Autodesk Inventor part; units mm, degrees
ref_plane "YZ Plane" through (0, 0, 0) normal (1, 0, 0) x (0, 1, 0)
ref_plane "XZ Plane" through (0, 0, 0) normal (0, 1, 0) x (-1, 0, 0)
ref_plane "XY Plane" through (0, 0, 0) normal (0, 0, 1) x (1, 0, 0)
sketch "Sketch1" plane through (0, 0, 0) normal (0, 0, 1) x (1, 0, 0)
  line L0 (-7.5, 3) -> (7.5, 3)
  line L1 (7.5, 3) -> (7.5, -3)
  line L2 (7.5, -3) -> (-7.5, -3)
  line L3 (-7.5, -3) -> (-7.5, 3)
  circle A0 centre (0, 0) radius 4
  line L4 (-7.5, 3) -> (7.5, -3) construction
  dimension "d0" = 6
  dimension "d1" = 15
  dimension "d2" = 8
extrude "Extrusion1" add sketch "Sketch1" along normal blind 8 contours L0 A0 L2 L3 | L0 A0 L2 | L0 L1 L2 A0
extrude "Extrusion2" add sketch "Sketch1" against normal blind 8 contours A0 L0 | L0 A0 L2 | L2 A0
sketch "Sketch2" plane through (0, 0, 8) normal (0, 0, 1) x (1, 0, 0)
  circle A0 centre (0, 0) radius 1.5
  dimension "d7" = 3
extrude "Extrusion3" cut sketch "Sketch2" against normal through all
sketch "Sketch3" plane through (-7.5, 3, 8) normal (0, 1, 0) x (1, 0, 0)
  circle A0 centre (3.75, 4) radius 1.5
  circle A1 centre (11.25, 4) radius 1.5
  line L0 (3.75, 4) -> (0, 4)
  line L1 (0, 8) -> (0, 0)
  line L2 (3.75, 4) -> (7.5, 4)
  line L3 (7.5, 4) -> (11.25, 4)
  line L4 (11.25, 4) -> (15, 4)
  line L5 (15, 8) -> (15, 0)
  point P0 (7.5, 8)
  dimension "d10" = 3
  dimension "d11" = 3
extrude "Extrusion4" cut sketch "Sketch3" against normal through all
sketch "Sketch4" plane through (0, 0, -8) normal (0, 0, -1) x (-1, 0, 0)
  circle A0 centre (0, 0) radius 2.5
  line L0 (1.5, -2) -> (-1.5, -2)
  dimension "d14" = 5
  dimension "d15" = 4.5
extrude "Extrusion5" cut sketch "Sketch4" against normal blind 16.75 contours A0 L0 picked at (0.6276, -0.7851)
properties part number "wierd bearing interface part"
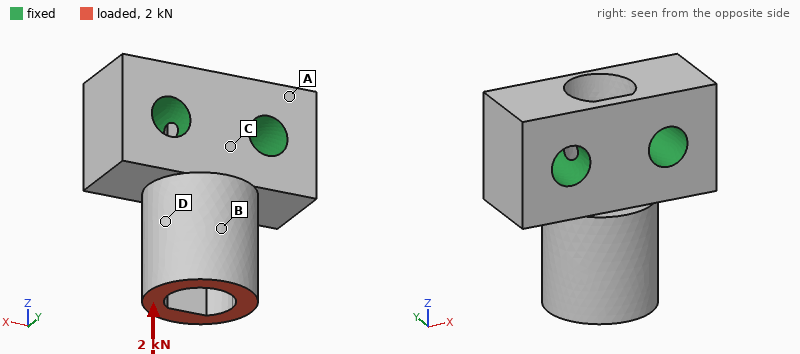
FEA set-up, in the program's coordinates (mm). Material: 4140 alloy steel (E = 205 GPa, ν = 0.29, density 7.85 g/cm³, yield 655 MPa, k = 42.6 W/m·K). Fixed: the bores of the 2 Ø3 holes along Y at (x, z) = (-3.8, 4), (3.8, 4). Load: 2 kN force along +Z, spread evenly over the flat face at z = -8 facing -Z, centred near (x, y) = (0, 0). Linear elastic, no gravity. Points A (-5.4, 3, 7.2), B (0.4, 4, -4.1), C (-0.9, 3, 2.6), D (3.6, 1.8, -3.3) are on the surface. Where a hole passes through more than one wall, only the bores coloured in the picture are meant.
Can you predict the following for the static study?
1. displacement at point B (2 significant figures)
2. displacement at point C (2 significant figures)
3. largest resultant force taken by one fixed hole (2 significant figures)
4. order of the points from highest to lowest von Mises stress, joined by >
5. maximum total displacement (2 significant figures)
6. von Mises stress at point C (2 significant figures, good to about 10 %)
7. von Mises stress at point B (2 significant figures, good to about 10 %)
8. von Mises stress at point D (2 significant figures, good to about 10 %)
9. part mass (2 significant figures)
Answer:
2.5 µm
0.65 µm
1.0 kN
D > B > C > A
3.6 µm
44 MPa
56 MPa
69 MPa
5.8 g
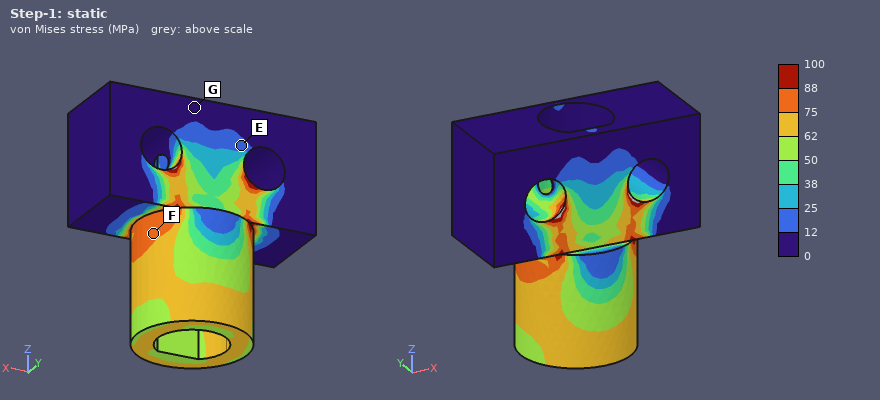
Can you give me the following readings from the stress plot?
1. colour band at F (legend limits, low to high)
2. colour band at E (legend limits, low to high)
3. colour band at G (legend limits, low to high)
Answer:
75 to 88 MPa
12 to 25 MPa
0 to 12 MPa
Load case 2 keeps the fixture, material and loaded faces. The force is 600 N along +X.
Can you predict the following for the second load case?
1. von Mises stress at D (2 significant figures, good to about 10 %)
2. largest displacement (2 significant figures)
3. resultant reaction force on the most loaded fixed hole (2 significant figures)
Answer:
61 MPa
10.0 µm
870 N
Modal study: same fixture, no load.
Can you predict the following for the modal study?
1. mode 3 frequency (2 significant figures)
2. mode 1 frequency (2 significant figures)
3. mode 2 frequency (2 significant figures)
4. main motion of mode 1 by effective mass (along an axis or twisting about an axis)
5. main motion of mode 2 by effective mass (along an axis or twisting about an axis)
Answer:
76 kHz
35 kHz
49 kHz
along Y
along X
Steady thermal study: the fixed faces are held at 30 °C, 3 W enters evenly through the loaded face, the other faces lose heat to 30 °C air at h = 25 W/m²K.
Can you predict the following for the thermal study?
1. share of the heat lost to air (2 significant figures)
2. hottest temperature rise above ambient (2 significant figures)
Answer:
4.3 %
23 K
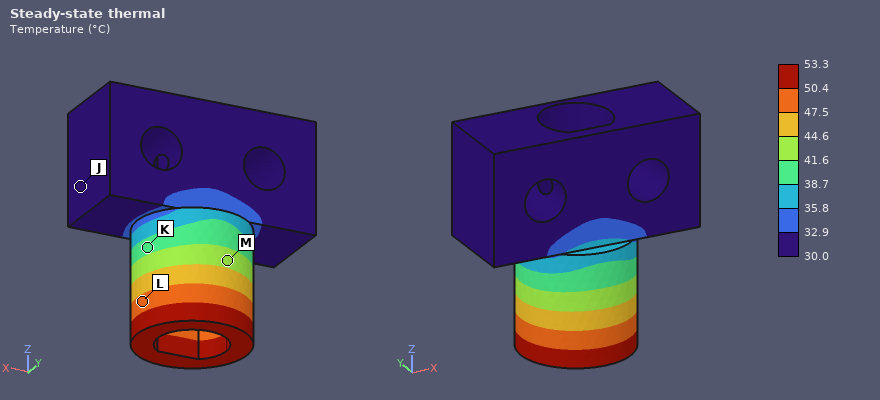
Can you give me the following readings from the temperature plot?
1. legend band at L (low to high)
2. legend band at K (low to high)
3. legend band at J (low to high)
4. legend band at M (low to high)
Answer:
47.5 to 50.4 °C
38.7 to 41.6 °C
30.0 to 32.9 °C
41.6 to 44.6 °C
